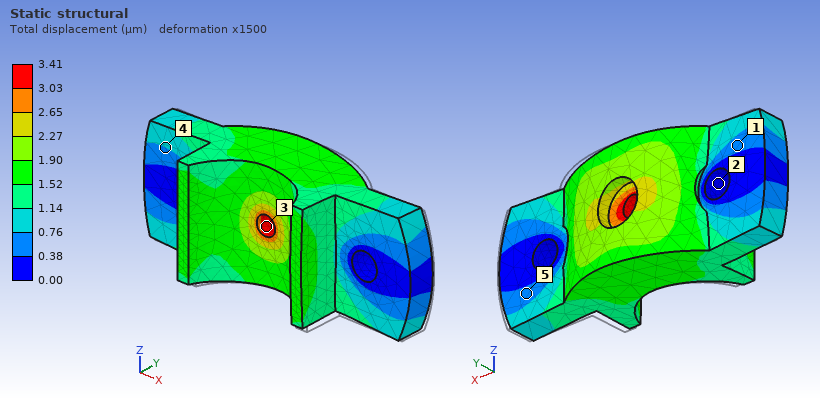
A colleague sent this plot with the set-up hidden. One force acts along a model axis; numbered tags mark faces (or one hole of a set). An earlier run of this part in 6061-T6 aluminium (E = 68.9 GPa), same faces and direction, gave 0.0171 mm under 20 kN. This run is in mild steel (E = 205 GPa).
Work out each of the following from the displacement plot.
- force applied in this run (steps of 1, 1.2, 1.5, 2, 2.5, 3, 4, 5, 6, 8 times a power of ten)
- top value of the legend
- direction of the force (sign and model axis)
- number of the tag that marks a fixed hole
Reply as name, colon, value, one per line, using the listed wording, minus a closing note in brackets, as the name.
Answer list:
force applied in this run: 12 kN
top value of the legend: 3.41 µm
direction of the force: -X
number of the tag that marks a fixed hole: 2
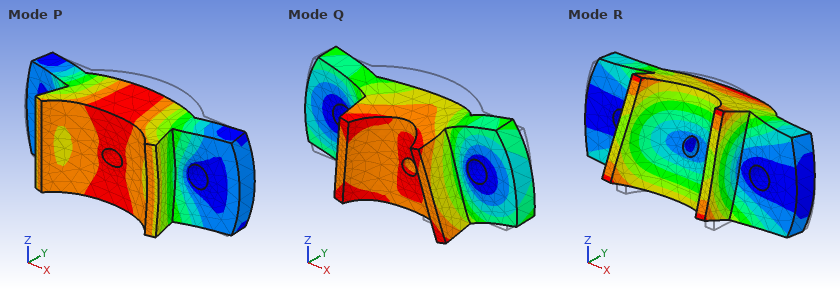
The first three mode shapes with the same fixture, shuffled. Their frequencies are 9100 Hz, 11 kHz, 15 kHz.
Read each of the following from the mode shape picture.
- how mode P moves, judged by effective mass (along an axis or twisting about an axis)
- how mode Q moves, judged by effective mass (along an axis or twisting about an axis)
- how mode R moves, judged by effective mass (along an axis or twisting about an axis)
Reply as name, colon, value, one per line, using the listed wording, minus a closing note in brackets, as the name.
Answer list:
how mode P moves, judged by effective mass: along Y
how mode Q moves, judged by effective mass: along Z
how mode R moves, judged by effective mass: twisting about X
